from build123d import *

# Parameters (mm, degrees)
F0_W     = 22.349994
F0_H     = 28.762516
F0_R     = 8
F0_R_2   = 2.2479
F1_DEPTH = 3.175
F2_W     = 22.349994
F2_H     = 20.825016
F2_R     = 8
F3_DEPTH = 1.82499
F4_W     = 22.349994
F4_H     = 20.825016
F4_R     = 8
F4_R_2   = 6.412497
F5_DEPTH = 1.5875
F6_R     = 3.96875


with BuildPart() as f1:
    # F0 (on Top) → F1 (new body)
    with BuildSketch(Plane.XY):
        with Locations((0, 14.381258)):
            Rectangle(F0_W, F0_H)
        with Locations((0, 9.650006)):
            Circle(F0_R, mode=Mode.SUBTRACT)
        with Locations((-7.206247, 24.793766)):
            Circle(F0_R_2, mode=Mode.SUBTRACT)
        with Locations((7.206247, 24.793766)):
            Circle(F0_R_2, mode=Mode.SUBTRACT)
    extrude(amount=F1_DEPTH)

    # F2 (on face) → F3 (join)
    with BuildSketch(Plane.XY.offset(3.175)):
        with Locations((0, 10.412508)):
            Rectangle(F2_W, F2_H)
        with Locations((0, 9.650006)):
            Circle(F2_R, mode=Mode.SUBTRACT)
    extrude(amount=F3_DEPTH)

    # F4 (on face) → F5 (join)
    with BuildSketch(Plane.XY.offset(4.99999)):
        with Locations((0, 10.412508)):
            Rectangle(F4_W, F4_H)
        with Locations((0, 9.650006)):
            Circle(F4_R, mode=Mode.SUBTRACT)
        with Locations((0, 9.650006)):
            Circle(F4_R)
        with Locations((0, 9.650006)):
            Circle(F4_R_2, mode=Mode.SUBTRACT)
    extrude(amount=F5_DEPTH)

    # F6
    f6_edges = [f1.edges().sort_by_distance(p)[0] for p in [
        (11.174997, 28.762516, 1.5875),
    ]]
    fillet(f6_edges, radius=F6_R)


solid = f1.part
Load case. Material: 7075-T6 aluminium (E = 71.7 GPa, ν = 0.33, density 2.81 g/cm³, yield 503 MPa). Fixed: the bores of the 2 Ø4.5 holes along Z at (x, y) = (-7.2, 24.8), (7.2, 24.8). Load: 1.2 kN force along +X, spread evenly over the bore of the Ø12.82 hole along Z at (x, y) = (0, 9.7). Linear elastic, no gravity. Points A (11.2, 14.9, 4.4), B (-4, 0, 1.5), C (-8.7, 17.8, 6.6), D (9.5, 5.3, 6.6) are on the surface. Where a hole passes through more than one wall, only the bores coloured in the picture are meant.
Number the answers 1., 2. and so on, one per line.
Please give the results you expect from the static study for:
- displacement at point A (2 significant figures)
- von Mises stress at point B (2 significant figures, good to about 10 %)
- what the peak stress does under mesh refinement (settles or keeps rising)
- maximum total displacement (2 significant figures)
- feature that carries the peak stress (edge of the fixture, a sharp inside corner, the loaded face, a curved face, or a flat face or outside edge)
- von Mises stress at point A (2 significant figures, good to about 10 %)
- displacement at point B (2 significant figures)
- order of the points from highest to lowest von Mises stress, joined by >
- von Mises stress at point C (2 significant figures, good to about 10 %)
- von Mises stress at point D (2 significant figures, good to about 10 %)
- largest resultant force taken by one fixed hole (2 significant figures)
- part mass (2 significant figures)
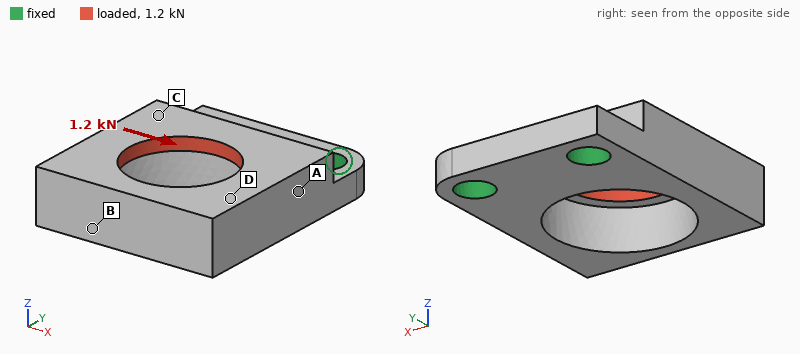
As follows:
1. 17 µm
2. 41 MPa
3. keeps rising
4. 59 µm
5. edge of the fixture
6. 62 MPa
7. 51 µm
8. A > B > D > C
9. 13 MPa
10. 22 MPa
11. 1.2 kN
12. 6.5 g
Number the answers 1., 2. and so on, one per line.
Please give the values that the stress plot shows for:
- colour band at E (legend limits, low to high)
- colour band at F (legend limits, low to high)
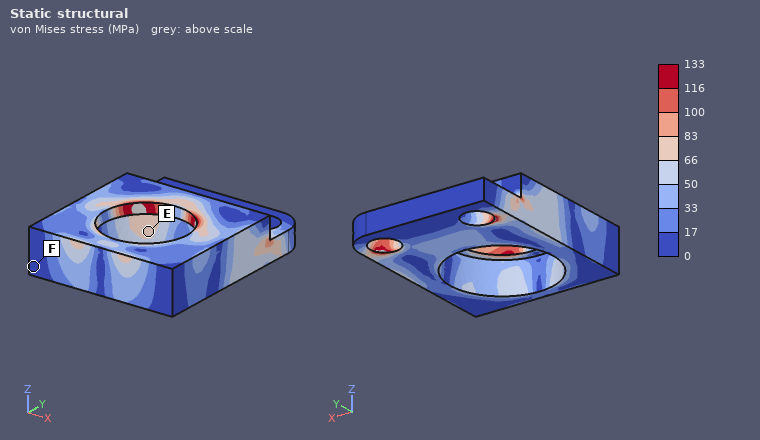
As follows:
1. 66 to 83 MPa
2. 0 to 17 MPa
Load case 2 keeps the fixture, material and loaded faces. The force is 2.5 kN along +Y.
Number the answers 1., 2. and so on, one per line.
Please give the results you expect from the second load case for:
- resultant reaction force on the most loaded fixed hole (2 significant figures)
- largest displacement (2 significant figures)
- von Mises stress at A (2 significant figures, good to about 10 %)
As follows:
1. 1.3 kN
2. 0.27 mm
3. 49 MPa
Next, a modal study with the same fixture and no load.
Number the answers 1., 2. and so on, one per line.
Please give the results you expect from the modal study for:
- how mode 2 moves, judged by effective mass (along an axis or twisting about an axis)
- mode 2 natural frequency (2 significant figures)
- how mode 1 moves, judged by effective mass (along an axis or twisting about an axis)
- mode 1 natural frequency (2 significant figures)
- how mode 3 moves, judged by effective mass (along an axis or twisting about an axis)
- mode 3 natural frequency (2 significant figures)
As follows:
1. along X
2. 10 kHz
3. along Z
4. 4900 Hz
5. along X
6. 14 kHz
